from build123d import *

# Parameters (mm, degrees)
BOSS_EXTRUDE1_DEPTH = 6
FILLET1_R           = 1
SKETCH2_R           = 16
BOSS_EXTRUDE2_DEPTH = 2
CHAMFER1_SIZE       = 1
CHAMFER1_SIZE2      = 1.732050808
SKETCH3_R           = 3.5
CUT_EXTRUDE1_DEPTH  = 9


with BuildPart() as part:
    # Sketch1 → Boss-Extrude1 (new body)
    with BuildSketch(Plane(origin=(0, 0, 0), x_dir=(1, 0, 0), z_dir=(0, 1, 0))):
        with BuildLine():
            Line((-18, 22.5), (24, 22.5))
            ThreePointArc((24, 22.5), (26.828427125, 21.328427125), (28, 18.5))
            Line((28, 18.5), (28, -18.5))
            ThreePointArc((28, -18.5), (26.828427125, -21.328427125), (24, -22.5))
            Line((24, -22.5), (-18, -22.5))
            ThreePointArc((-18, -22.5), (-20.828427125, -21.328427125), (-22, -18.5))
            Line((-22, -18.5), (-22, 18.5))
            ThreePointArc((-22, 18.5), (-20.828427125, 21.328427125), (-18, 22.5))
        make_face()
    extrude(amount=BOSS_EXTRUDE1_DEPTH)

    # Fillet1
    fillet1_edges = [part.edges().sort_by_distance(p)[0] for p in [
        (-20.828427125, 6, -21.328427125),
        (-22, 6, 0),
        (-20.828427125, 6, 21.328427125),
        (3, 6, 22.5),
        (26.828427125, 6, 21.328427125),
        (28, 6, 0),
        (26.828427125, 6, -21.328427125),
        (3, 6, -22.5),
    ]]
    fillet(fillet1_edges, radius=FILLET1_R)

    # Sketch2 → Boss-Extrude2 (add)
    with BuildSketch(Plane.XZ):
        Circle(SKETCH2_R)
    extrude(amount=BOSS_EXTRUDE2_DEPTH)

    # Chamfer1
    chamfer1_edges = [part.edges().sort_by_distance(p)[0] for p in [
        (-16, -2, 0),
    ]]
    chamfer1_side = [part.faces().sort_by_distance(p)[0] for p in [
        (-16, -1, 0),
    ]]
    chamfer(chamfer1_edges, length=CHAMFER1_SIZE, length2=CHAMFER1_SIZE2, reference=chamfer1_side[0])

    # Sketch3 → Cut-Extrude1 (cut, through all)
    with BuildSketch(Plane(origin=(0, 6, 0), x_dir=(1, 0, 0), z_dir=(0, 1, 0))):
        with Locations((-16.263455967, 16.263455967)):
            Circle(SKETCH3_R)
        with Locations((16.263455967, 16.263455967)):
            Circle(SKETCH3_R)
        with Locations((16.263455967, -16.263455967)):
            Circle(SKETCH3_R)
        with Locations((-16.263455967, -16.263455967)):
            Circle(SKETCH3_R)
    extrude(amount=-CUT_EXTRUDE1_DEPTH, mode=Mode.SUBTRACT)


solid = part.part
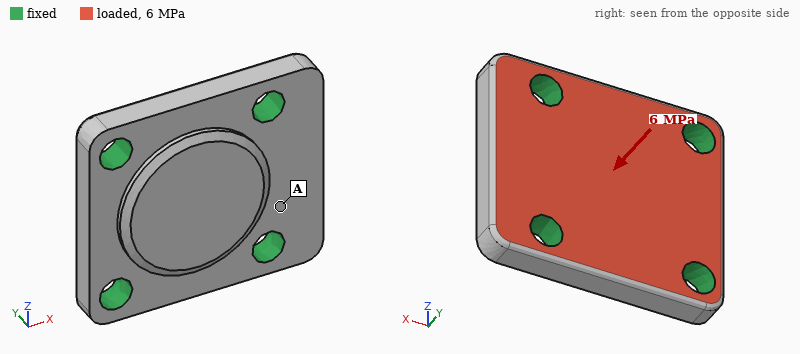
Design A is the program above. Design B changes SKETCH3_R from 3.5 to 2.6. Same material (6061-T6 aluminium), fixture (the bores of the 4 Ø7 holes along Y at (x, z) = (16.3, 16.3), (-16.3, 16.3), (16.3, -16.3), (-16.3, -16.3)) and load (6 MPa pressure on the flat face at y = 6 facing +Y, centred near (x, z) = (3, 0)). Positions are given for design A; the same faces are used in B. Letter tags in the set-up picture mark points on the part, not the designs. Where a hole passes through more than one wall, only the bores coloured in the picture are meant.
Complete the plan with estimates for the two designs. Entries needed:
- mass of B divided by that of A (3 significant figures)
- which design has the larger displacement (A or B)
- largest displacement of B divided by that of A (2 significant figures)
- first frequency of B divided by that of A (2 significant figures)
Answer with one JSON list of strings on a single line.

["1.03", "B", "1.3", "0.89"]
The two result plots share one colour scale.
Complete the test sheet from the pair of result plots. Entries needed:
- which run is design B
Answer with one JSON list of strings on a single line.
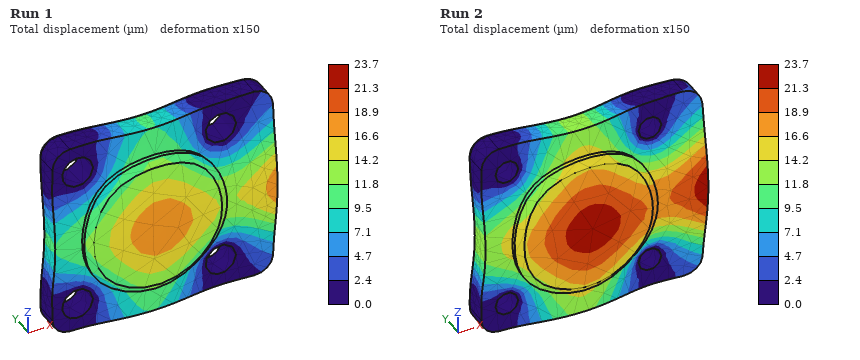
["Run 2"]
